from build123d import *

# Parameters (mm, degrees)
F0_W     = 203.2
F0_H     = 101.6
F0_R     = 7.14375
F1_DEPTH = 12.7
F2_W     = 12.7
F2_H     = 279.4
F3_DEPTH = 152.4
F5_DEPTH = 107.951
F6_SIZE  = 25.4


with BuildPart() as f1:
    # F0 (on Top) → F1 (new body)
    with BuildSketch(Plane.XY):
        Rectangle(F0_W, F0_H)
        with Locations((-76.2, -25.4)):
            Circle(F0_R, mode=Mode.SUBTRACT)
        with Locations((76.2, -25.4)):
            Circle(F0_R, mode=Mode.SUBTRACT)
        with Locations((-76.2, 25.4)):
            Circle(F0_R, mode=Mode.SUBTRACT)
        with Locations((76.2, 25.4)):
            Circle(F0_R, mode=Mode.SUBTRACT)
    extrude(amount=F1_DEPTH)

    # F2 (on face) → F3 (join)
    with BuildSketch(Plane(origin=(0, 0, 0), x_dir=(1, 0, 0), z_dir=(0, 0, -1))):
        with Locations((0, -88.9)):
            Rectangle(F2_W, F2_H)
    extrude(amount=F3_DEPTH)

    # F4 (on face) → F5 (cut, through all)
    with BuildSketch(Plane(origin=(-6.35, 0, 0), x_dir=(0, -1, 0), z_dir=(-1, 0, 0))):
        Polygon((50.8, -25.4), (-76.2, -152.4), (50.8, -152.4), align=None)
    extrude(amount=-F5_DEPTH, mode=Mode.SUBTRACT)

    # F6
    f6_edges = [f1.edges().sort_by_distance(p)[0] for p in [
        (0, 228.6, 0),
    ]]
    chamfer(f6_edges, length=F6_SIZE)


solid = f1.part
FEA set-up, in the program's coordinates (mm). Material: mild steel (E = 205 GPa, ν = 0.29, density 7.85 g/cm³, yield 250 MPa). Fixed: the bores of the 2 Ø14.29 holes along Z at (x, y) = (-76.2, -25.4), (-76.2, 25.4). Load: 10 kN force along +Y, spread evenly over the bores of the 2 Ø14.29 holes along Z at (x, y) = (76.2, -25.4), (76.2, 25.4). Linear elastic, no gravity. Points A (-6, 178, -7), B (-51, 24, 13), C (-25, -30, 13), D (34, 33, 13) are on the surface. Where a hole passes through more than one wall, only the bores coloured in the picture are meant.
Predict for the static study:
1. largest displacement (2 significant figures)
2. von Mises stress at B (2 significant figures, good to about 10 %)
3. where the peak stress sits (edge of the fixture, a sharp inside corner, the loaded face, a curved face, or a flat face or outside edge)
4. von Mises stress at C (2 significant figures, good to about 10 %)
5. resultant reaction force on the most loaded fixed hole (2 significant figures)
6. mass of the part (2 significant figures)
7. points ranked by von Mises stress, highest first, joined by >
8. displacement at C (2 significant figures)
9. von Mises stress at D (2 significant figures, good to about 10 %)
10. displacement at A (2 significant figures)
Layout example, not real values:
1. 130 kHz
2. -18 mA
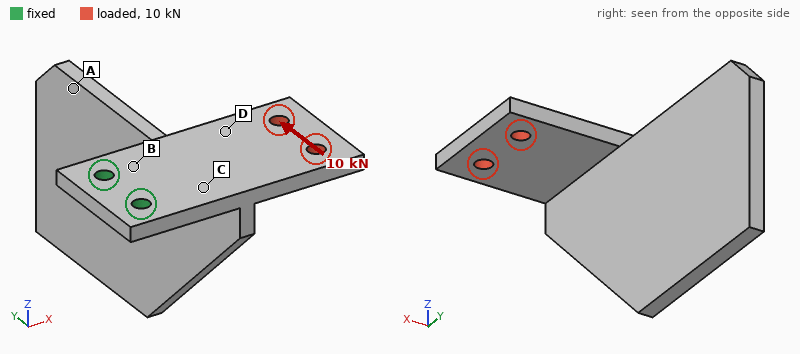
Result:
1. 0.12 mm
2. 44 MPa
3. edge of the fixture
4. 31 MPa
5. 25 kN
6. 5.4 kg
7. B > C > D > A
8. 0.021 mm
9. 17 MPa
10. 0.093 mm
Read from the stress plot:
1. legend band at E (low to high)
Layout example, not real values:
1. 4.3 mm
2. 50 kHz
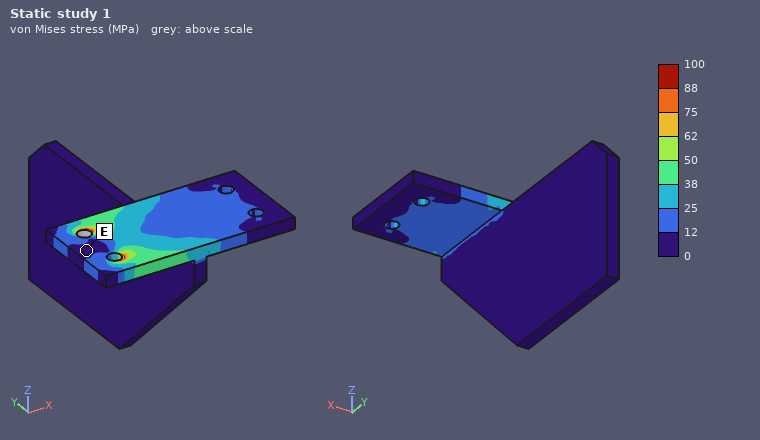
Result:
1. 0 to 12 MPa
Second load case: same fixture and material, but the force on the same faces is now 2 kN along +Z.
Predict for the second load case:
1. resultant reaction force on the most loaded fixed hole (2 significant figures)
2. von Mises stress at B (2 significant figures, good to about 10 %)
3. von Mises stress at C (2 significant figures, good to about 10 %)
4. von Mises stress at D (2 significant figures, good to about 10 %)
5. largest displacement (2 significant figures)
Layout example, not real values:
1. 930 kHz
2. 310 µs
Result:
1. 1.0 kN
2. 86 MPa
3. 68 MPa
4. 30 MPa
5. 0.75 mm
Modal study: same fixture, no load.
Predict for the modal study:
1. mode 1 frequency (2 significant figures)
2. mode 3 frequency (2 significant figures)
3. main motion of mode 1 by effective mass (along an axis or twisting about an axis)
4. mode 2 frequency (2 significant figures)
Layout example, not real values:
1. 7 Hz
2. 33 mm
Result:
1. 130 Hz
2. 310 Hz
3. along X
4. 200 Hz
